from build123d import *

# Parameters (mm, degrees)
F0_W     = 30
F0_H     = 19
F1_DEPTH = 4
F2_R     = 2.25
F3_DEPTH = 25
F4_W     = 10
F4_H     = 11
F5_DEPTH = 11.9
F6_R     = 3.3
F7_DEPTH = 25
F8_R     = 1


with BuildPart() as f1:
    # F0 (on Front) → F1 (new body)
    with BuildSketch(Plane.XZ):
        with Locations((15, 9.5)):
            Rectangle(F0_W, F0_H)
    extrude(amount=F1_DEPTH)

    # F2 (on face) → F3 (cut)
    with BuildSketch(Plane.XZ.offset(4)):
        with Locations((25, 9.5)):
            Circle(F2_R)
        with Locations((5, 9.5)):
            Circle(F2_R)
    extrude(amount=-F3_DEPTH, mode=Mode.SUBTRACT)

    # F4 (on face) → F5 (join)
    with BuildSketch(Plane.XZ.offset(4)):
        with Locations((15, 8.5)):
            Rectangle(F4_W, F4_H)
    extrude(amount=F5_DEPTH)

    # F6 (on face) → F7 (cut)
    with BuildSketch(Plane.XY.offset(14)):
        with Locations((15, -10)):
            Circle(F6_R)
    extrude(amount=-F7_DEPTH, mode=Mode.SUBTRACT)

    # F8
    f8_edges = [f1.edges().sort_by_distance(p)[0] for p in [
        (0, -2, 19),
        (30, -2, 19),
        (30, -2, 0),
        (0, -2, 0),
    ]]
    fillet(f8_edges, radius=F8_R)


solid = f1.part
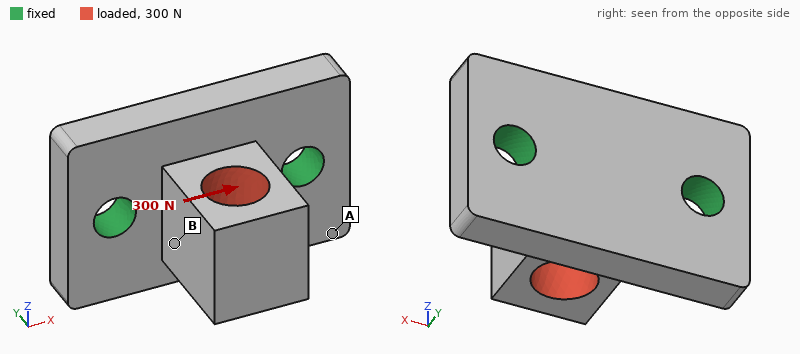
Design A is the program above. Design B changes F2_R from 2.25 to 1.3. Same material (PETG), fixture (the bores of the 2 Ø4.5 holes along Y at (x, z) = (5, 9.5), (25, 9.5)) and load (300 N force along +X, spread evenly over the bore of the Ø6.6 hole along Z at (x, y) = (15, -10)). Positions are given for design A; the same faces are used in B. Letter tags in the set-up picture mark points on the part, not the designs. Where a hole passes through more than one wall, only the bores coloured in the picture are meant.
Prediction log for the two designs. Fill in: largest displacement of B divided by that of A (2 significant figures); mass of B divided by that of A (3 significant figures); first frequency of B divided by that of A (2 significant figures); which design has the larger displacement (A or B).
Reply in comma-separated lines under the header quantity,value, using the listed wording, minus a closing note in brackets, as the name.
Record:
quantity,value
largest displacement of B divided by that of A,1.1
mass of B divided by that of A,1.03
first frequency of B divided by that of A,0.82
which design has the larger displacement,B
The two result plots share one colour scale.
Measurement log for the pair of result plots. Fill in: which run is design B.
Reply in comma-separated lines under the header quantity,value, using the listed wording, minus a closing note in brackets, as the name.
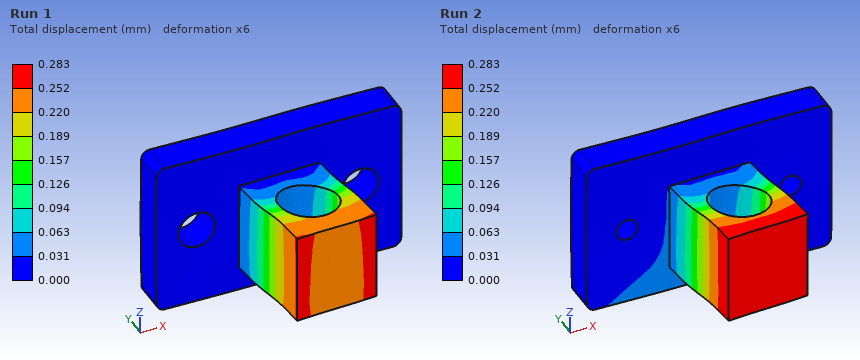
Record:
quantity,value
which run is design B,Run 2
